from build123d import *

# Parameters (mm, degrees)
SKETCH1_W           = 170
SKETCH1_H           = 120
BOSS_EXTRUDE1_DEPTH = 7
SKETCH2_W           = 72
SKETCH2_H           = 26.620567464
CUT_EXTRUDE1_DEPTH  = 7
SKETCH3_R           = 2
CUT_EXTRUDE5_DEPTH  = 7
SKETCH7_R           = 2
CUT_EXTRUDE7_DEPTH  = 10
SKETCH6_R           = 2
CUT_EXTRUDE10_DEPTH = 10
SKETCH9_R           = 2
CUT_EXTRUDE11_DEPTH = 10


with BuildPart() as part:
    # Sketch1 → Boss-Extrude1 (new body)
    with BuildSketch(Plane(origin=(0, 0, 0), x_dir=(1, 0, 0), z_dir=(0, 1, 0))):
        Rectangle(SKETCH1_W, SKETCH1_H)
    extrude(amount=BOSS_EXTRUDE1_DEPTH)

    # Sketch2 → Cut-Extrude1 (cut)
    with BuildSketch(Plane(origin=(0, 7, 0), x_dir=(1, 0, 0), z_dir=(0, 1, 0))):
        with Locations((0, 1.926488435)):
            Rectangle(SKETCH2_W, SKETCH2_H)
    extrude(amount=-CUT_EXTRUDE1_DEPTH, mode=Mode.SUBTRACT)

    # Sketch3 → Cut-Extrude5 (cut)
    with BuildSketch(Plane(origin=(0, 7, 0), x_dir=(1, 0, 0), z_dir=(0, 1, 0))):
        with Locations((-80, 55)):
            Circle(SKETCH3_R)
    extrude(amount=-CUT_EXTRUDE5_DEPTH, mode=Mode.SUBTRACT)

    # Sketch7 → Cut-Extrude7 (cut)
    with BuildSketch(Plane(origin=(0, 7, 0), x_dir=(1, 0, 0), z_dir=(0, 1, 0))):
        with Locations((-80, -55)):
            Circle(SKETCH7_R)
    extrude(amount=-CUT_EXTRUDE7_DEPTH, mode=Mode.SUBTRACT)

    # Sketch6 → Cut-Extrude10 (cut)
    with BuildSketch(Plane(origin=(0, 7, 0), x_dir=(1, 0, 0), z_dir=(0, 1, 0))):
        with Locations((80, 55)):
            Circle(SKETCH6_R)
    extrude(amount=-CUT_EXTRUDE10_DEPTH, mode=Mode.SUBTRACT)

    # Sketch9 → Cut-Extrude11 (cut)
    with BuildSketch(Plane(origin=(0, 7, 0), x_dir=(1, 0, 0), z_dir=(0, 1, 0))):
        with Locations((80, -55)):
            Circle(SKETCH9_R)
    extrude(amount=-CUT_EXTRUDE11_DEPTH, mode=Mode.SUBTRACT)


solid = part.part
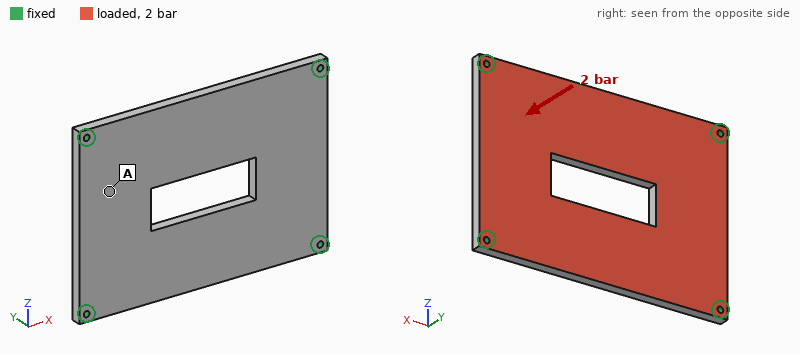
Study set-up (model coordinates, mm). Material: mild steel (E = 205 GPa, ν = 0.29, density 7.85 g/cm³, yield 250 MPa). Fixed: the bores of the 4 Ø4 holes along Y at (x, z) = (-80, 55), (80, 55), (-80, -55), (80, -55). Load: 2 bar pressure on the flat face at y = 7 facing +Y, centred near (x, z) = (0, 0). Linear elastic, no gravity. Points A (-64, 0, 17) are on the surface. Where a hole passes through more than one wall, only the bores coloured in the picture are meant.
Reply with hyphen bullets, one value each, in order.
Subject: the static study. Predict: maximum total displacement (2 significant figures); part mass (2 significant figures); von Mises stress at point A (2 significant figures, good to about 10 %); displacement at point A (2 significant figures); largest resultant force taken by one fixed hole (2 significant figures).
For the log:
- 0.14 mm
- 1.0 kg
- 21 MPa
- 0.051 mm
- 920 N
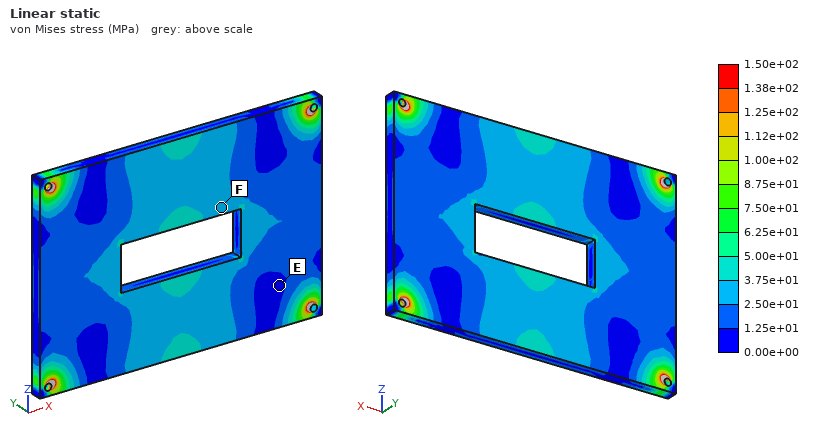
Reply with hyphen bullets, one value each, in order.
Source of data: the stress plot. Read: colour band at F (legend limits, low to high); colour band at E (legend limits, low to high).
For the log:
- 2.50e+01 to 3.75e+01 MPa
- 0.00e+00 to 1.25e+01 MPa
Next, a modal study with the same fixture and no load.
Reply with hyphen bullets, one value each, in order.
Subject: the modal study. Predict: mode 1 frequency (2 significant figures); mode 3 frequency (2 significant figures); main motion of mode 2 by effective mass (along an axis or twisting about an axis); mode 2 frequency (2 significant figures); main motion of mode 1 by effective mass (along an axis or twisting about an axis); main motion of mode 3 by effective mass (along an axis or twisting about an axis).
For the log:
- 1000 Hz
- 2400 Hz
- twisting about X
- 1600 Hz
- along Y
- twisting about Z
